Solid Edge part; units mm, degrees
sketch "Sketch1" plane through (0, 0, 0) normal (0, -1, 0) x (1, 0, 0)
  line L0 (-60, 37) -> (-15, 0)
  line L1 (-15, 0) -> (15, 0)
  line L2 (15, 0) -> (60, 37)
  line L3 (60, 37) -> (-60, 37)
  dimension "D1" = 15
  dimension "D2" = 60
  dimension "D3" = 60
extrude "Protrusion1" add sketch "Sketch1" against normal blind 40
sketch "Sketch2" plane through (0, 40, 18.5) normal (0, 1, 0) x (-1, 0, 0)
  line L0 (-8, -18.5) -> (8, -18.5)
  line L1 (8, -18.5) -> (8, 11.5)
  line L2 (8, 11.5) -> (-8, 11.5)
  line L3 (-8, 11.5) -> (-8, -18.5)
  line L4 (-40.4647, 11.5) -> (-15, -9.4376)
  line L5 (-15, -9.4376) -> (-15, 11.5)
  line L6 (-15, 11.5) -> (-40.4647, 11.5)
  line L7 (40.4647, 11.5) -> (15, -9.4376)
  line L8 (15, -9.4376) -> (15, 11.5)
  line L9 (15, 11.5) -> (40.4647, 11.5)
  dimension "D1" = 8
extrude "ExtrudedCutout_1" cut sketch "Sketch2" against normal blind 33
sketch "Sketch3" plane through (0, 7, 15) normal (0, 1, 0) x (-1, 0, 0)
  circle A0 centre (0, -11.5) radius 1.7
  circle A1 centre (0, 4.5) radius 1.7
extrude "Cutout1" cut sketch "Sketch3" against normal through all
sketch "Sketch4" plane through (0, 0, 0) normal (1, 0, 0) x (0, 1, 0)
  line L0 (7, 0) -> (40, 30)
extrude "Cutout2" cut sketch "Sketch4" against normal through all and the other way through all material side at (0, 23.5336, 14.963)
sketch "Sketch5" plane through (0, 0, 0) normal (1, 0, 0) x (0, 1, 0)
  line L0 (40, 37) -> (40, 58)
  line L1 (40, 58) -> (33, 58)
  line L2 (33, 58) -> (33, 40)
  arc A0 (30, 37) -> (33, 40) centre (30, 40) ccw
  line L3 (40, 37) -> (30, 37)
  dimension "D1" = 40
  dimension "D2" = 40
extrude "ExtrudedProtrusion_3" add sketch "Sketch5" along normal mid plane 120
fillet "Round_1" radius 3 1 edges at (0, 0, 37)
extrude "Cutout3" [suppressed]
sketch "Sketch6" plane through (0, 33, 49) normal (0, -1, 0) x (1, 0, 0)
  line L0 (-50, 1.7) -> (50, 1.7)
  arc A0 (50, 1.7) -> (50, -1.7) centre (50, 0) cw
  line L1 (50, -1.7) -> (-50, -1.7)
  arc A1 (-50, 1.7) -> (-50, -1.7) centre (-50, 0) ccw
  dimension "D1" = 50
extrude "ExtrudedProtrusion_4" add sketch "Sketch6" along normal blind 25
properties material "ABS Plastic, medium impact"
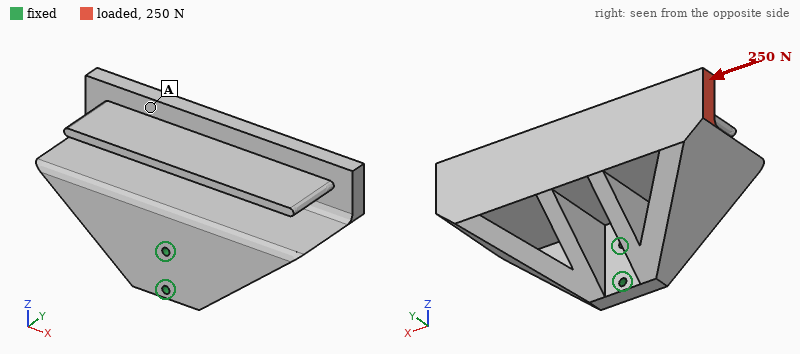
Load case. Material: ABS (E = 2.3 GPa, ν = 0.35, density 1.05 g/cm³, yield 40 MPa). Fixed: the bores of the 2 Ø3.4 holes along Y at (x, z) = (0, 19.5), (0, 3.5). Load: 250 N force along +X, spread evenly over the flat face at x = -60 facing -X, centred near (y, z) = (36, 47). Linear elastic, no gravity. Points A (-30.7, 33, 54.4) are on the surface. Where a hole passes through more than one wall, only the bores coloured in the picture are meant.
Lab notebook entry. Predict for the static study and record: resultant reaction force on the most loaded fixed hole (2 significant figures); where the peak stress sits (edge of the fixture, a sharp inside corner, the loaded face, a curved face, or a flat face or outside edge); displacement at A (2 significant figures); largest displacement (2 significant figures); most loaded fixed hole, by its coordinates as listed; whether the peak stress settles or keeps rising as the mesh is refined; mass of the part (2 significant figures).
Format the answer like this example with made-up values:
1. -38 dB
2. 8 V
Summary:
1. 620 N
2. edge of the fixture
3. 0.92 mm
4. 1.5 mm
5. (0, 19.5)
6. keeps rising
7. 93 g
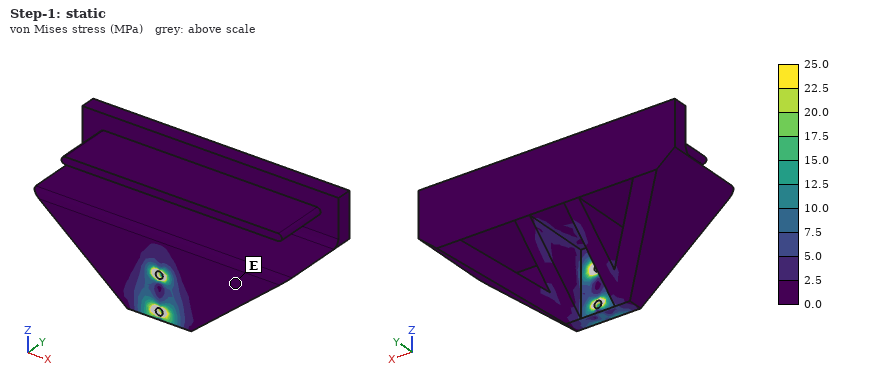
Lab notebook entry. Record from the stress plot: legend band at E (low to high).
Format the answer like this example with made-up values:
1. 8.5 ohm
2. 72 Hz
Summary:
1. 0.0 to 2.5 MPa
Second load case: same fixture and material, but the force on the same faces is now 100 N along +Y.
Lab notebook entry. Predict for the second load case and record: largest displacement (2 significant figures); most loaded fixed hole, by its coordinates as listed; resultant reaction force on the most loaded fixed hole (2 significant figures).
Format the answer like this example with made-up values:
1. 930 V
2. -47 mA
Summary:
1. 1.5 mm
2. (0, 19.5)
3. 220 N
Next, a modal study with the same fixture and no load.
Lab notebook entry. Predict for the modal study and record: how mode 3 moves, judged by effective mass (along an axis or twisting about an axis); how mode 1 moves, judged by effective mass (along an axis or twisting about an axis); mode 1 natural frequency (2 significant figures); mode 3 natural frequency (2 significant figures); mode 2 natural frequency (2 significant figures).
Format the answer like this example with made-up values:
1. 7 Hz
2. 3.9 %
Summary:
1. along X
2. along X
3. 280 Hz
4. 690 Hz
5. 520 Hz
